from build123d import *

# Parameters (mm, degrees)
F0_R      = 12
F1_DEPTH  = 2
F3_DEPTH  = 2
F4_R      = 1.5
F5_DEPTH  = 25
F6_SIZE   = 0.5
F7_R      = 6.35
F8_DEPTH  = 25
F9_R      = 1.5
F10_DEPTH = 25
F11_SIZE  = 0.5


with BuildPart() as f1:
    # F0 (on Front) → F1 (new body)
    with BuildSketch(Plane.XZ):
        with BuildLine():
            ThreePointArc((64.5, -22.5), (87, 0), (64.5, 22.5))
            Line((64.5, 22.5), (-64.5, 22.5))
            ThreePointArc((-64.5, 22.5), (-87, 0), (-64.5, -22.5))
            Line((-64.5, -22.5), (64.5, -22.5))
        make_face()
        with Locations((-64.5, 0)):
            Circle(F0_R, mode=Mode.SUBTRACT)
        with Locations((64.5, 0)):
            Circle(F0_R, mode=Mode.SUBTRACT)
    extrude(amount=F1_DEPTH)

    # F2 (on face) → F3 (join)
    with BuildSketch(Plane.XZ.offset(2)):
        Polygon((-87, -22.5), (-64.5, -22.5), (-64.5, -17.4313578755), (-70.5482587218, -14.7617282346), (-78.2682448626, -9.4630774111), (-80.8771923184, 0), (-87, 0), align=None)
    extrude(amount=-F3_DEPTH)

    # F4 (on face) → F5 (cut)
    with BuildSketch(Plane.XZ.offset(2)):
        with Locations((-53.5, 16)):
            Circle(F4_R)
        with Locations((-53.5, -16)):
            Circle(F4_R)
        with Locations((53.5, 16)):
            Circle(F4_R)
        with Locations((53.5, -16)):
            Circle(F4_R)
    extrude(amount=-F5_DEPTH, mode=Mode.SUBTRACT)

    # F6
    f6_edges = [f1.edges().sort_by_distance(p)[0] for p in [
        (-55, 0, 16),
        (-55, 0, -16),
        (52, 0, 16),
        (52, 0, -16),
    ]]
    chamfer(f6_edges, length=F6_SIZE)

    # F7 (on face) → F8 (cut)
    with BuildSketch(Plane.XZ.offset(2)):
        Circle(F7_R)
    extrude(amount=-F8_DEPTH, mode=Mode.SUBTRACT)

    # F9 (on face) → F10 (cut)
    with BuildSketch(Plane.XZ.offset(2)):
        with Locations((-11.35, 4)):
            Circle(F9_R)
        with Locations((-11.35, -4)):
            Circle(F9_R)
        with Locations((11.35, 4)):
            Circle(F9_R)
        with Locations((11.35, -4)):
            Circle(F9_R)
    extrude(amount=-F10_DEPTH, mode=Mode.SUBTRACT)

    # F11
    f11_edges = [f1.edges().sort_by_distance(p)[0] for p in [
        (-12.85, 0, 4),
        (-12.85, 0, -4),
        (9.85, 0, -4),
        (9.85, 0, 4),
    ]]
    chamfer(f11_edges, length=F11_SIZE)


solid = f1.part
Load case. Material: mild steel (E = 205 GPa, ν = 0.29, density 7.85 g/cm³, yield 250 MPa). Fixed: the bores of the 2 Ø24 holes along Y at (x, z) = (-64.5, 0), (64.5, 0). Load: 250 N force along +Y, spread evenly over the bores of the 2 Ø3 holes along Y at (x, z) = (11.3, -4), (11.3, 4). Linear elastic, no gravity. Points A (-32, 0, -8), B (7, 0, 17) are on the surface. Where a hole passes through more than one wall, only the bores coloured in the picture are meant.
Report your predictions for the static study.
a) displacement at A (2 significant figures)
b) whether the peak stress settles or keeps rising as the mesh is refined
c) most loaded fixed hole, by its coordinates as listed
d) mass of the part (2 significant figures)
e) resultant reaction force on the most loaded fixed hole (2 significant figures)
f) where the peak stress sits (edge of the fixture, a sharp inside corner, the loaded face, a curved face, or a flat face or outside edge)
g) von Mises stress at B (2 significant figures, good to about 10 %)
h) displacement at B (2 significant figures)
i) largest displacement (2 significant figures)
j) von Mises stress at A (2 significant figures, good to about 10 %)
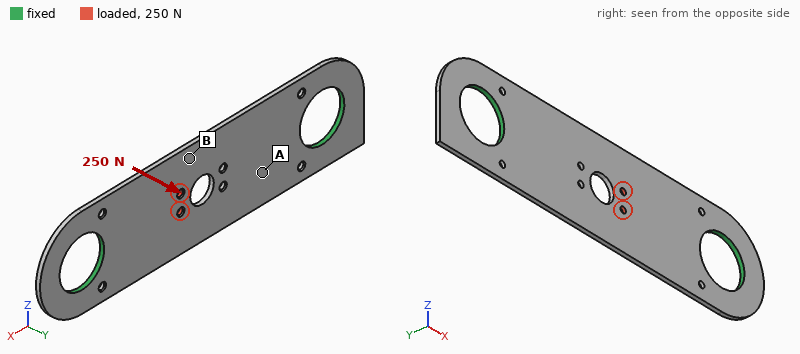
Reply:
0.083 mm
keeps rising
(64.5, 0)
100 g
160 N
a sharp inside corner
95 MPa
0.26 mm
0.29 mm
24 MPa
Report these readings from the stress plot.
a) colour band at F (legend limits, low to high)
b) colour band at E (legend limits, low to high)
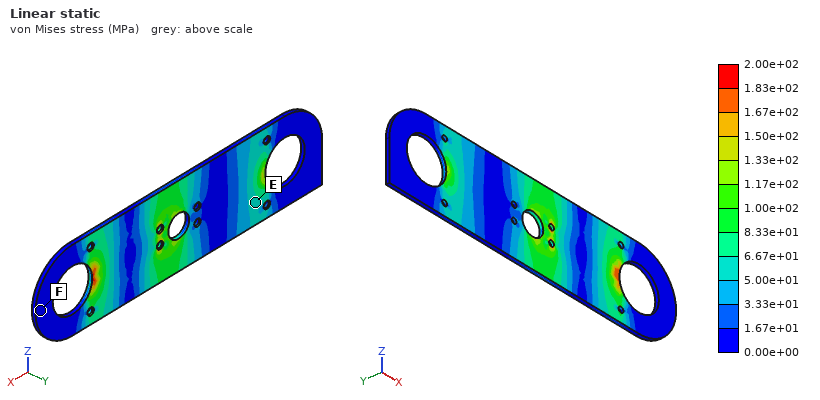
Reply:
0.00e+00 to 1.67e+01 MPa
5.00e+01 to 6.67e+01 MPa
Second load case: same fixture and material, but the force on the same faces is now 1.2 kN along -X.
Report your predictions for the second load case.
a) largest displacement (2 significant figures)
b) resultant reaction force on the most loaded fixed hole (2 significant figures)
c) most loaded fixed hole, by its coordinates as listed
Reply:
8.4 µm
790 N
(64.5, 0)
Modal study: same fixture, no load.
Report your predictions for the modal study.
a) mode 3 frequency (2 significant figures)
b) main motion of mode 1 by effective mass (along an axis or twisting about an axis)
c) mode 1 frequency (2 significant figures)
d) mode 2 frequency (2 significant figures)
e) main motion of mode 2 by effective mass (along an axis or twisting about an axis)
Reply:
2300 Hz
along Y
880 Hz
1500 Hz
twisting about X
